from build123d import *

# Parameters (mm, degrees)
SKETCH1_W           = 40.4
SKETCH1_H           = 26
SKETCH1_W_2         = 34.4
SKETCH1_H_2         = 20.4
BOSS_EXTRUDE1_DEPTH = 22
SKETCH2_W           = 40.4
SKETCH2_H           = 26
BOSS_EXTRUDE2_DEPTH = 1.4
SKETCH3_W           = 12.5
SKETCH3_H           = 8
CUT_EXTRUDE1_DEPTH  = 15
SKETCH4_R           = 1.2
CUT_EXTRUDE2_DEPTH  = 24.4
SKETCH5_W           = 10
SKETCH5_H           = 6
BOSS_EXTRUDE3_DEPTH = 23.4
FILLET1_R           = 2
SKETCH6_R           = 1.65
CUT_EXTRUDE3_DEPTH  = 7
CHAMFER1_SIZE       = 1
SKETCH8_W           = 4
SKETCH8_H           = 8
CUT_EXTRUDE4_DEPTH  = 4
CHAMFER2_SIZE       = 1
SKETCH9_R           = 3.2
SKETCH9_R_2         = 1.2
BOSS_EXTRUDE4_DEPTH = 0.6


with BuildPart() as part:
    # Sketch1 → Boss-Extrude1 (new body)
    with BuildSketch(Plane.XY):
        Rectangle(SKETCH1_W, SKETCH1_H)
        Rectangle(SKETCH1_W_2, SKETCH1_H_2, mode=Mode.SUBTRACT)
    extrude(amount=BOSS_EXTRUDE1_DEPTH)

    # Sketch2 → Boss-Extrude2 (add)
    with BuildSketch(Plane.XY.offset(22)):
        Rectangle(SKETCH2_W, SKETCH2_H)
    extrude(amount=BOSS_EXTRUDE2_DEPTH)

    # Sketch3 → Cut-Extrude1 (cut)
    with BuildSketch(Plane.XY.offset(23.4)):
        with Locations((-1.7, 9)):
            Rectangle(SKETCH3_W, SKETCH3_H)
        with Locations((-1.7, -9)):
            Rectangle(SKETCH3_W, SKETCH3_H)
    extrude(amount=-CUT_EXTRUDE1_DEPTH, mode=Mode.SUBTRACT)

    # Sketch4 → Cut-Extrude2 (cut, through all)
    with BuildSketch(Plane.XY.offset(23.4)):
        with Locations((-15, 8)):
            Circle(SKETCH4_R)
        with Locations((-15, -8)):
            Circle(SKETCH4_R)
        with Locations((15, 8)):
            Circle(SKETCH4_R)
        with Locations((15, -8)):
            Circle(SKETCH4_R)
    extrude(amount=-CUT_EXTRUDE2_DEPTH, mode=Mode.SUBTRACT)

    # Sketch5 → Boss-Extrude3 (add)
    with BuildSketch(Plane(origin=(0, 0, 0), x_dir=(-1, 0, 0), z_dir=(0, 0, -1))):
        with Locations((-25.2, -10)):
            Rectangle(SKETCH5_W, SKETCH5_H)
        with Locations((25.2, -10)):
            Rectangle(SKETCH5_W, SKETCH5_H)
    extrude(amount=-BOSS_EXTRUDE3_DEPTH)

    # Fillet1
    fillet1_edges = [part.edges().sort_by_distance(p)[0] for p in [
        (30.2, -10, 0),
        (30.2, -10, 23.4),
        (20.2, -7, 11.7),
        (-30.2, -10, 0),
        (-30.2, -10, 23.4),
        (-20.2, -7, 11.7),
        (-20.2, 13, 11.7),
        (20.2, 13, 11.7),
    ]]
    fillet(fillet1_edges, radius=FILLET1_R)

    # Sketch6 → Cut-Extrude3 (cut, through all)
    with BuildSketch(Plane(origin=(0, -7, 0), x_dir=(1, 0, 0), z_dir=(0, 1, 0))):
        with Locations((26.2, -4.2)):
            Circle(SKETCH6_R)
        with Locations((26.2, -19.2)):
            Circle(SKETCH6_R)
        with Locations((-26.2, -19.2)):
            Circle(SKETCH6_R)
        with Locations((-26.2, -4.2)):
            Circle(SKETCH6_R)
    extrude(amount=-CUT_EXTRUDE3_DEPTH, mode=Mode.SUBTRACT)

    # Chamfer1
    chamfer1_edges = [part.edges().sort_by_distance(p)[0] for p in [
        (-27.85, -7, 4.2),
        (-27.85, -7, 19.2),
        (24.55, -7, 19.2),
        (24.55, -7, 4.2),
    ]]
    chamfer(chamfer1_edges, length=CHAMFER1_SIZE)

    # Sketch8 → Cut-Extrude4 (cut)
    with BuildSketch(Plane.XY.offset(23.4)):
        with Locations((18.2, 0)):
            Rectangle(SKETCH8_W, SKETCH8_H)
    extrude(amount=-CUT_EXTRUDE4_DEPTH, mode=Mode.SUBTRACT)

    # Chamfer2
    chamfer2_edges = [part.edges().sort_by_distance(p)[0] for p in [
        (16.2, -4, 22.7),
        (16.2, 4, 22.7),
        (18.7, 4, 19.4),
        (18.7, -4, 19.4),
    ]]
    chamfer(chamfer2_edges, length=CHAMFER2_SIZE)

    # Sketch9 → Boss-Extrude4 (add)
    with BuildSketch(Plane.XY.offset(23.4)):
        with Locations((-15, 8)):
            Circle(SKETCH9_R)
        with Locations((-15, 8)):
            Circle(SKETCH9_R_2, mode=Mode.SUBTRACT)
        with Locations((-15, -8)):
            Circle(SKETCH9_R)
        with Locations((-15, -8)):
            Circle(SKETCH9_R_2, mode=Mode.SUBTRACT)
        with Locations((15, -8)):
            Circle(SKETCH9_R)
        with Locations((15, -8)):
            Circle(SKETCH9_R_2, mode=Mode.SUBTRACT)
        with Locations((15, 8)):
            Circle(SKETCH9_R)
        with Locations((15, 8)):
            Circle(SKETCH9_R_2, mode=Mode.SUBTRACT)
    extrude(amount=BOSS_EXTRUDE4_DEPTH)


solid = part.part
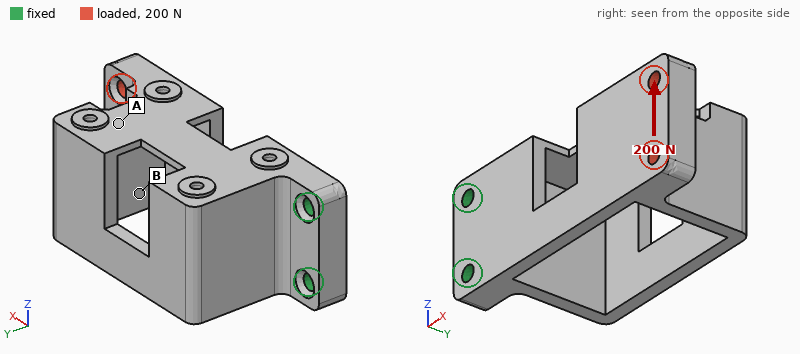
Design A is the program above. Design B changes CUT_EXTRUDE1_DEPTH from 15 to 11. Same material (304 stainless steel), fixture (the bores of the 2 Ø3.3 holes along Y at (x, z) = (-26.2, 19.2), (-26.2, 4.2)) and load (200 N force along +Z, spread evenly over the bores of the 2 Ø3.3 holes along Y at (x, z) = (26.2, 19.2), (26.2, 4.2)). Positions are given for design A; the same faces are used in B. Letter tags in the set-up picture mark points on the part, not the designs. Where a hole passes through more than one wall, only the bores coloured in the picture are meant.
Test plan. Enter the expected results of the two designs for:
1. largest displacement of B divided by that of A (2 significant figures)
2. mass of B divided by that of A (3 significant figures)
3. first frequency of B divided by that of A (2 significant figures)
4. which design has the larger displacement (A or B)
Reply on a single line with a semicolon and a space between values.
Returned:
0.73; 1.03; 1.0; A
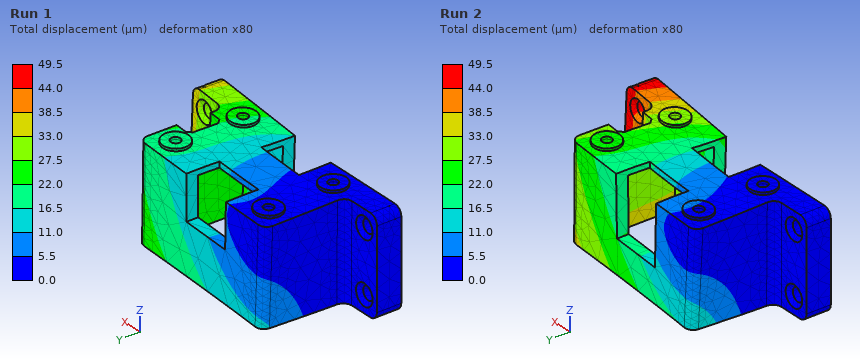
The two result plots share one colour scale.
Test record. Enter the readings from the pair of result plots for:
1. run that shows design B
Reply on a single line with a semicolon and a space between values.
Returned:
Run 1
